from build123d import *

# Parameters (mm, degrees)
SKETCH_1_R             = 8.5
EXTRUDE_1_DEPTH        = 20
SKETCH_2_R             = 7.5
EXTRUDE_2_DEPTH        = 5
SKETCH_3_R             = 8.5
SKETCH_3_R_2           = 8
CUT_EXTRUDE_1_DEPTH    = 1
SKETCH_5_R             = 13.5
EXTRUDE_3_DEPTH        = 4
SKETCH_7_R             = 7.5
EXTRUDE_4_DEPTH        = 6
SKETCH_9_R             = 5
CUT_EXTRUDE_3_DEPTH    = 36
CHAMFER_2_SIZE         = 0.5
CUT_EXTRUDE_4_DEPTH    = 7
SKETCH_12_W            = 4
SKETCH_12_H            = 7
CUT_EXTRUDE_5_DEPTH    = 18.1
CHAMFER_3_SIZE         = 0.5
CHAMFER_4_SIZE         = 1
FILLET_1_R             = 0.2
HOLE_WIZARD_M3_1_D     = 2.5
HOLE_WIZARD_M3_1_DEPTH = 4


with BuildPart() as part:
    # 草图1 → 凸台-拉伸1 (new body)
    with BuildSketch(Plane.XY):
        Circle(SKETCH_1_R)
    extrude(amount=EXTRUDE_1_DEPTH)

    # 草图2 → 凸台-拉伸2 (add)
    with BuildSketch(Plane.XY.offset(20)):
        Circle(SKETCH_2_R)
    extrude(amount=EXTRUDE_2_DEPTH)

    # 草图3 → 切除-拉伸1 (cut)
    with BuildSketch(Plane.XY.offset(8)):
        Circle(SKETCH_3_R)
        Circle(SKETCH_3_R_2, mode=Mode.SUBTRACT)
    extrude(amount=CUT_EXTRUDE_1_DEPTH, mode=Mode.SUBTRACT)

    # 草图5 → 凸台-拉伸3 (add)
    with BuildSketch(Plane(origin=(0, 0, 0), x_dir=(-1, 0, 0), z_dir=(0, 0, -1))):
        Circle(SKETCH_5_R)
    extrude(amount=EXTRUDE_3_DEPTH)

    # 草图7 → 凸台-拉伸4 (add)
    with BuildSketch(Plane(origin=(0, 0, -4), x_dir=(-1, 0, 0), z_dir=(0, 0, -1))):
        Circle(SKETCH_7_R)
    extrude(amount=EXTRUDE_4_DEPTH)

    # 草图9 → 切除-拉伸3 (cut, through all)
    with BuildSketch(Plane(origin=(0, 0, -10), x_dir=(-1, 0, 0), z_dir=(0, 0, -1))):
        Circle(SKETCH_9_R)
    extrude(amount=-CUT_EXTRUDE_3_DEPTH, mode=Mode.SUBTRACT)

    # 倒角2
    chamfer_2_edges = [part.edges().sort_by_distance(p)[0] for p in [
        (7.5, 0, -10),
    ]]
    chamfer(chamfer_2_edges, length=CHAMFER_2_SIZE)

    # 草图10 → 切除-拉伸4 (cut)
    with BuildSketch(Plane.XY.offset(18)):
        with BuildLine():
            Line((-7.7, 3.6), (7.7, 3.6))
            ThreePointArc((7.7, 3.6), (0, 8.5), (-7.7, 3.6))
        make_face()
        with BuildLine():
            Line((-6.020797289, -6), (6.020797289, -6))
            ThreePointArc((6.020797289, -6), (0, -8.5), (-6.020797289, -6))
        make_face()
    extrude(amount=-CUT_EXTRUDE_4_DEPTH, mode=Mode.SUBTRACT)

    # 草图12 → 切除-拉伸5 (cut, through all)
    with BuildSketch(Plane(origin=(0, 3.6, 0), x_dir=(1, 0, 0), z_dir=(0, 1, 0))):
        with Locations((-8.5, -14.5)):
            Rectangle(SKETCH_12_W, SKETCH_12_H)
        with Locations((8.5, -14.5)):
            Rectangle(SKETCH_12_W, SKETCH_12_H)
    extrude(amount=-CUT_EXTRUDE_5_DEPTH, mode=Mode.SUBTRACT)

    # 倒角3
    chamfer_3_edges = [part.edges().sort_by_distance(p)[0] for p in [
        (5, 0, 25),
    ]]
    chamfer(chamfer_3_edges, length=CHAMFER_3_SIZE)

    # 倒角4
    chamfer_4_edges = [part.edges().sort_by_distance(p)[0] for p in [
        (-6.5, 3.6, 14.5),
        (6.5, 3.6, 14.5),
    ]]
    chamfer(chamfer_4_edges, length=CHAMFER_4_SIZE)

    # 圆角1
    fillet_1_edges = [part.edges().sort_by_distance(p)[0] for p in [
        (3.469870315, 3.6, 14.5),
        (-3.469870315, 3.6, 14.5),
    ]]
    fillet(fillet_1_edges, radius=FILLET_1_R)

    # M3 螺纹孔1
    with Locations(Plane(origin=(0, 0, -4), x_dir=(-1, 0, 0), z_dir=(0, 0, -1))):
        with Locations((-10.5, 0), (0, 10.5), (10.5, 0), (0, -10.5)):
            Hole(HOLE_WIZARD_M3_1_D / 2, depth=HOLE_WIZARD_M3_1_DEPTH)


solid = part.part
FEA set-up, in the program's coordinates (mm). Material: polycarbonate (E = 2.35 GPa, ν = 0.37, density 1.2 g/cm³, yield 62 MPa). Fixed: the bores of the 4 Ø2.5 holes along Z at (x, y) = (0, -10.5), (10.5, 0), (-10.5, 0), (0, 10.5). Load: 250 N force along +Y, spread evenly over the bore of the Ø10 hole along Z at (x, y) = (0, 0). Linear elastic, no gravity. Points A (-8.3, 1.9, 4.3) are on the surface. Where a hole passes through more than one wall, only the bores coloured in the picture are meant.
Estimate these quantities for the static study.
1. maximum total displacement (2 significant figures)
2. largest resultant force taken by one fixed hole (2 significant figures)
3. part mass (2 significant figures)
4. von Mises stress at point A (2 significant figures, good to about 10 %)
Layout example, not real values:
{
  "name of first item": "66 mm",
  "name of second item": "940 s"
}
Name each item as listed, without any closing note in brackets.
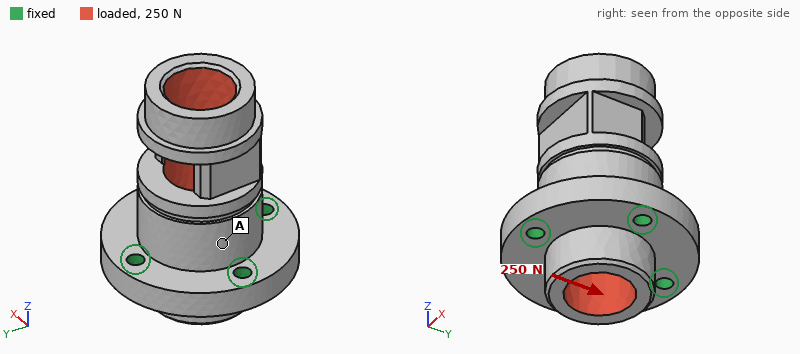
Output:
{
  "maximum total displacement": "0.18 mm",
  "largest resultant force taken by one fixed hole": "130 N",
  "part mass": "6.3 g",
  "von Mises stress at point A": "2.4 MPa"
}
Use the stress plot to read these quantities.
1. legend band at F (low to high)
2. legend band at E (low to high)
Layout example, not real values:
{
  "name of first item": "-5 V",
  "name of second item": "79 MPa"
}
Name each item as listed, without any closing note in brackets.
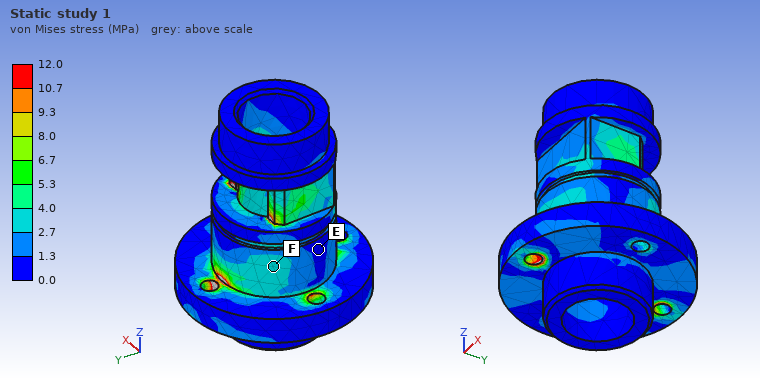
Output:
{
  "legend band at F": "2.7 to 4.0 MPa",
  "legend band at E": "0.0 to 1.3 MPa"
}
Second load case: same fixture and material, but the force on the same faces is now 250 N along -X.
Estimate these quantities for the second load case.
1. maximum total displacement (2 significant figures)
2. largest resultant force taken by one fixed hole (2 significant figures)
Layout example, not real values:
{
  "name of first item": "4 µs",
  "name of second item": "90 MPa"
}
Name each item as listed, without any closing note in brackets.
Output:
{
  "maximum total displacement": "0.24 mm",
  "largest resultant force taken by one fixed hole": "130 N"
}
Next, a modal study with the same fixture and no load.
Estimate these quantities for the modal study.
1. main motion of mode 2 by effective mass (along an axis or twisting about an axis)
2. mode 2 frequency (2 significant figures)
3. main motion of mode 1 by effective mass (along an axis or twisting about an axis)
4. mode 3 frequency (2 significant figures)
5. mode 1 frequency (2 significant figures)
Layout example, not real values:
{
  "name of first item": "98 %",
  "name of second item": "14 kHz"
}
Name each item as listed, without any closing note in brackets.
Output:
{
  "main motion of mode 2 by effective mass": "along Y",
  "mode 2 frequency": "3400 Hz",
  "main motion of mode 1 by effective mass": "along X",
  "mode 3 frequency": "6100 Hz",
  "mode 1 frequency": "3000 Hz"
}
